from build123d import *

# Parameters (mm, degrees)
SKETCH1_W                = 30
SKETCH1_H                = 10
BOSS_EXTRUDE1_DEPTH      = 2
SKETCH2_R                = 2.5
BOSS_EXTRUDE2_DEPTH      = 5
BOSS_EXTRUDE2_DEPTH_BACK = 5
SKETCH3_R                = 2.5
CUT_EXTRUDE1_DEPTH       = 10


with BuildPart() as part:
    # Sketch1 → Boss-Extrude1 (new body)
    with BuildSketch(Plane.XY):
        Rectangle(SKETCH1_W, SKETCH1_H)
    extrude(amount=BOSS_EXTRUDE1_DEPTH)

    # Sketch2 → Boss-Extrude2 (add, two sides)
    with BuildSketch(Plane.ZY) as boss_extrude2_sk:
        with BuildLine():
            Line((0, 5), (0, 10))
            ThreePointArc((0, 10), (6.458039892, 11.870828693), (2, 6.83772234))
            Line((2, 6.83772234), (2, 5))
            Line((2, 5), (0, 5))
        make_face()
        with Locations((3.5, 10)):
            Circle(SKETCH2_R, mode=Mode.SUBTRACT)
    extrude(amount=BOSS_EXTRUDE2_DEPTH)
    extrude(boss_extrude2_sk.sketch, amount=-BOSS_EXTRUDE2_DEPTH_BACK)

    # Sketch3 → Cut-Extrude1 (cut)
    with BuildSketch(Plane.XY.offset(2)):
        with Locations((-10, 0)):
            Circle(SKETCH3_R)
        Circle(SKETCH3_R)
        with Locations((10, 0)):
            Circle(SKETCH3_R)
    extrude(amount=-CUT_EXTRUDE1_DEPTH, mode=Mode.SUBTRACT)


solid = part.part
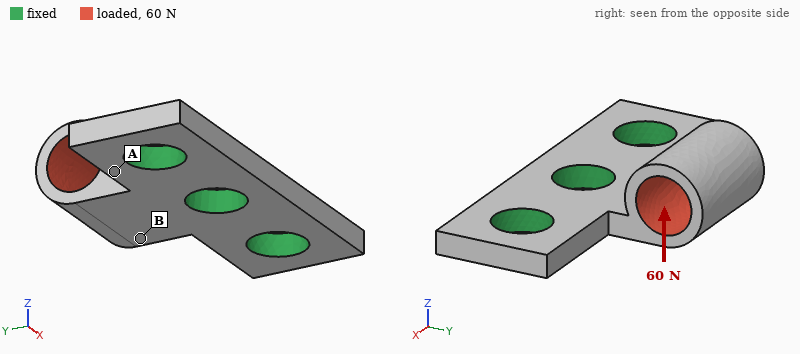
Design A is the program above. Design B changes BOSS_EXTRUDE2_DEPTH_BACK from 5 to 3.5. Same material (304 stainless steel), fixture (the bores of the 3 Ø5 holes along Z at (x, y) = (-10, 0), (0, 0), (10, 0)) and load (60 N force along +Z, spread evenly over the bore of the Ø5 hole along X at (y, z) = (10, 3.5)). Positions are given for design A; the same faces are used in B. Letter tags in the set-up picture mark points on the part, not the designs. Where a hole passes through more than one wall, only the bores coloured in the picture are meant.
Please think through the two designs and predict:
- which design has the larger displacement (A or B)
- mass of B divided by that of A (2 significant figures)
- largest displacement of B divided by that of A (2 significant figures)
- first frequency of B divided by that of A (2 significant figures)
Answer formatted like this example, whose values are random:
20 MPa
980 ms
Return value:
B
0.95
1.2
1.0
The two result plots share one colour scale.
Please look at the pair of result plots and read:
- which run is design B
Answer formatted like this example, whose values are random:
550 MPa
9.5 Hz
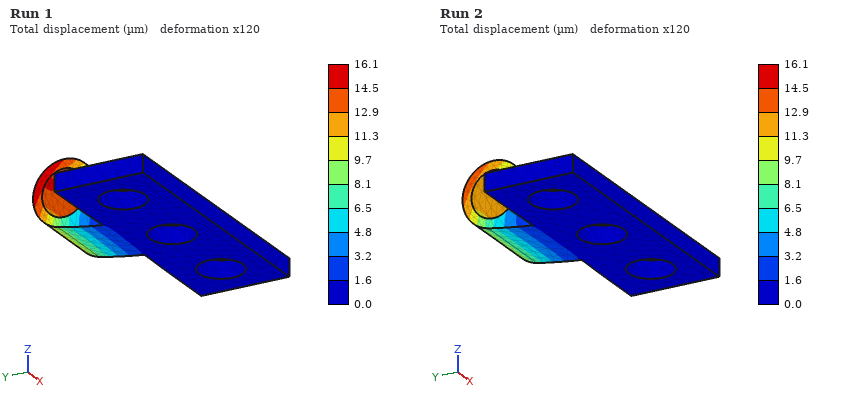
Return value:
Run 1
